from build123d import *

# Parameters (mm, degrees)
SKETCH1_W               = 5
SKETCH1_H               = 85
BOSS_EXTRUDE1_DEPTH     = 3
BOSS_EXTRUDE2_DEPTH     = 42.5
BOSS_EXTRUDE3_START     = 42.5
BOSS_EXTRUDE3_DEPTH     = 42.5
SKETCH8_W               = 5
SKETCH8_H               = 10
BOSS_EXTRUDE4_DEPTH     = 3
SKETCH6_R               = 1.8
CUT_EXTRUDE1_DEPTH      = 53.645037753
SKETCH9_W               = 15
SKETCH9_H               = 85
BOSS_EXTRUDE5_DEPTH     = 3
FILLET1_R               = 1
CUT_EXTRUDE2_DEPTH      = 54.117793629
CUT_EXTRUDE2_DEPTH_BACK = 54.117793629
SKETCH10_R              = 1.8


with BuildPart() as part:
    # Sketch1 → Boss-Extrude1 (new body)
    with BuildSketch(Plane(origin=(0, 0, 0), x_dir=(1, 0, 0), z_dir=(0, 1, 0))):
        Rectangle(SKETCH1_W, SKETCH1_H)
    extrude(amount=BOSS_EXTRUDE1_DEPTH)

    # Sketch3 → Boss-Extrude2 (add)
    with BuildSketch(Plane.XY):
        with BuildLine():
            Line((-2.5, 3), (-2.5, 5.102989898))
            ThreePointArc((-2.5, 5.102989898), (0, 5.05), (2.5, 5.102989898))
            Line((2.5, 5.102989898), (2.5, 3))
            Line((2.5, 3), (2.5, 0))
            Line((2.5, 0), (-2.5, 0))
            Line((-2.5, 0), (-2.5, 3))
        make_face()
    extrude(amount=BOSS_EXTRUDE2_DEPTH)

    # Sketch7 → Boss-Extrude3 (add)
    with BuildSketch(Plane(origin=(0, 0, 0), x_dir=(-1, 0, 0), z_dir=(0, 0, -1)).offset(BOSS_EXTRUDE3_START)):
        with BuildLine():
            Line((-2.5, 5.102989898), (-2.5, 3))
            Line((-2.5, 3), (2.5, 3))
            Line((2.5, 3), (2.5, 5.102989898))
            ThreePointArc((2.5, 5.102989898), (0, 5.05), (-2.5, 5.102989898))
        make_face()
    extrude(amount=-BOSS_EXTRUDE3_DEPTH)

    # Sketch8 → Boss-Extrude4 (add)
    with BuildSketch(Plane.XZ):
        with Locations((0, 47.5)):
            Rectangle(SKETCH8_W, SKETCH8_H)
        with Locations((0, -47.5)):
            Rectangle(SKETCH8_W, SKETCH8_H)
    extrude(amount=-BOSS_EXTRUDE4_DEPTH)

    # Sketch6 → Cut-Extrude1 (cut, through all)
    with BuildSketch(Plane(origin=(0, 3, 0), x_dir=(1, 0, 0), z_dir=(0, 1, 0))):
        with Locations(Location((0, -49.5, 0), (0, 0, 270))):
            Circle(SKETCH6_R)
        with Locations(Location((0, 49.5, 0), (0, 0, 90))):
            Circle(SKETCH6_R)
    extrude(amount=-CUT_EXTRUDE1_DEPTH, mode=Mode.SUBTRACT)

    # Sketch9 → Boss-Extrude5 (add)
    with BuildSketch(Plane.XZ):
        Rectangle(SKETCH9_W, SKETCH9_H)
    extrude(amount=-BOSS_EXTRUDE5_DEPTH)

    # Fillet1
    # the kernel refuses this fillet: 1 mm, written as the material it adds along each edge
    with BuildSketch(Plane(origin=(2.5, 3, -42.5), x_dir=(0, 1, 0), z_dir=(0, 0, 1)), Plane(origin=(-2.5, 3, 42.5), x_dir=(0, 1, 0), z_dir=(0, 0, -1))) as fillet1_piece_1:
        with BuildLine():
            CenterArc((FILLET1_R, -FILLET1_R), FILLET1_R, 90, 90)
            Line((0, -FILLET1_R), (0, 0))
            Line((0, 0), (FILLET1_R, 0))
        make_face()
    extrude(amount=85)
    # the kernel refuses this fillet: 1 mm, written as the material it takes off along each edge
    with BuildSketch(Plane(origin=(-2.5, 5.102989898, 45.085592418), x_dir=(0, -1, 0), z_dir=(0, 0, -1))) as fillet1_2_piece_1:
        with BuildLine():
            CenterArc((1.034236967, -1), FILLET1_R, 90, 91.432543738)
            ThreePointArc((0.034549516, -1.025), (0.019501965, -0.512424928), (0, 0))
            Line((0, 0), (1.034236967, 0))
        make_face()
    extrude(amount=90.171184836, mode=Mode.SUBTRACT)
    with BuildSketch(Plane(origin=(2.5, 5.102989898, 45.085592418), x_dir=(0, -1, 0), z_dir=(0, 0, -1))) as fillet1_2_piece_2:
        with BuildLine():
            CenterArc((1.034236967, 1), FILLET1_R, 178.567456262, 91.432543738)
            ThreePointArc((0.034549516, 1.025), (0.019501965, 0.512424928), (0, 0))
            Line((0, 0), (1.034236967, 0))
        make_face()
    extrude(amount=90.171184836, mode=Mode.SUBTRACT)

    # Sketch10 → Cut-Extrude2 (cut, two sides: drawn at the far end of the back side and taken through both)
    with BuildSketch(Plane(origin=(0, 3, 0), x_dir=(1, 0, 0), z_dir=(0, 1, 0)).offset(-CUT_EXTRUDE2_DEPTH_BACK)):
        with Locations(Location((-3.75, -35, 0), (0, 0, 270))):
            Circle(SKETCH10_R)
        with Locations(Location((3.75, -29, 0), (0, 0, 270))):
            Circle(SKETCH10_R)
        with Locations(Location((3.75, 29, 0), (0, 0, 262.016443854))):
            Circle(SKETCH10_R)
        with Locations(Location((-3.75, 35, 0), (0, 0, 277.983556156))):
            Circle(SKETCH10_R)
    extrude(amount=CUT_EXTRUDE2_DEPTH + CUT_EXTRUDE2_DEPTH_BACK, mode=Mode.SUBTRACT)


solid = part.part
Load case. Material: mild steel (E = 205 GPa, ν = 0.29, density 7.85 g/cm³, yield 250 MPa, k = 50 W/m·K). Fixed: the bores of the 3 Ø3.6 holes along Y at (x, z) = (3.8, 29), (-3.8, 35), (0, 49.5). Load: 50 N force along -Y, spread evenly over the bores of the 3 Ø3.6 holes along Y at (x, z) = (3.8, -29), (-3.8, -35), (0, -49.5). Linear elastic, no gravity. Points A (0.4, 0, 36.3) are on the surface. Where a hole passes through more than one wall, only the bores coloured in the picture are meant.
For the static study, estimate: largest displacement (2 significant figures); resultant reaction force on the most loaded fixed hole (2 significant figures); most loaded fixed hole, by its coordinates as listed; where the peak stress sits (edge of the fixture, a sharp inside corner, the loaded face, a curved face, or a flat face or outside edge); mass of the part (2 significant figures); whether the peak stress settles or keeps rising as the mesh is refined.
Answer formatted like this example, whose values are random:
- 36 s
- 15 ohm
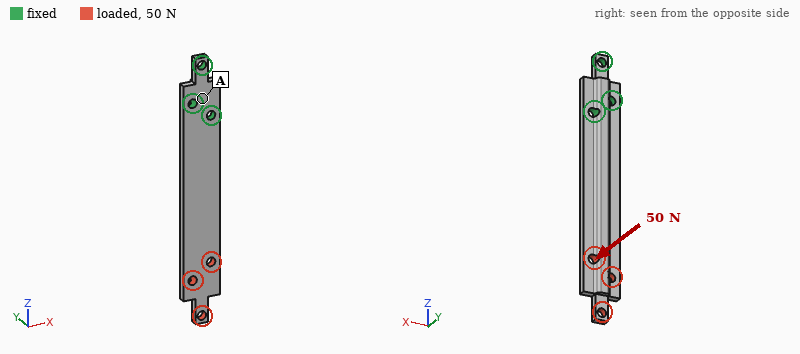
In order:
- 0.37 mm
- 190 N
- (3.8, 29)
- edge of the fixture
- 38 g
- keeps rising
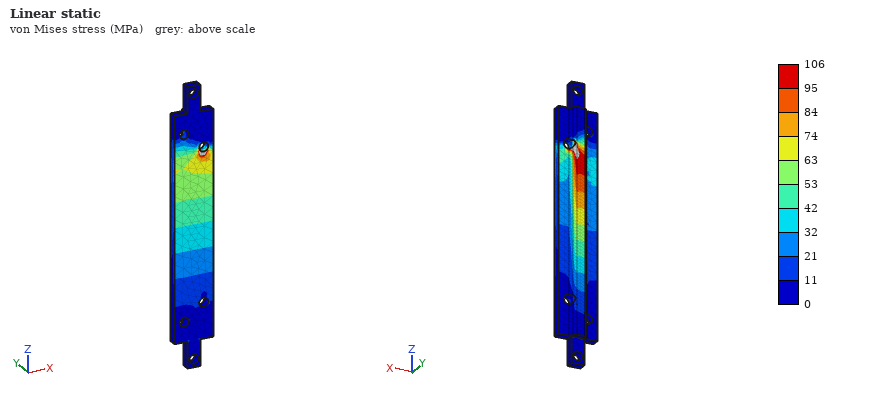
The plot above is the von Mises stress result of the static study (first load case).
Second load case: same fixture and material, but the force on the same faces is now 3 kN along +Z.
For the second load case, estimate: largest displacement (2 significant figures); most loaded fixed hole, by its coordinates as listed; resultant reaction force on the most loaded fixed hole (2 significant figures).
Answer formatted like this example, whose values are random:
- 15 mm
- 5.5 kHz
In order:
- 0.13 mm
- (3.8, 29)
- 1.7 kN
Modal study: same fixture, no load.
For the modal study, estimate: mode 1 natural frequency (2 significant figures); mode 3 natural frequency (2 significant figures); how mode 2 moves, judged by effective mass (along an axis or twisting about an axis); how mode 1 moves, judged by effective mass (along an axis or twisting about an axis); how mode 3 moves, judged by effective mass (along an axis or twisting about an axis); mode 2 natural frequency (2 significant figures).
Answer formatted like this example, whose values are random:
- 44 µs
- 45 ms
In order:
- 670 Hz
- 3900 Hz
- along X
- along Y
- along Y
- 2000 Hz
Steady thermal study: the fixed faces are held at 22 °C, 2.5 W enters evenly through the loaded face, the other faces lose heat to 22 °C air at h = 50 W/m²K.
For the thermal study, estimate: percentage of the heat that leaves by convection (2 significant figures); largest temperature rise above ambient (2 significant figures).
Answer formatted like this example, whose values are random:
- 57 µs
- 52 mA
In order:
- 73 %
- 34 K
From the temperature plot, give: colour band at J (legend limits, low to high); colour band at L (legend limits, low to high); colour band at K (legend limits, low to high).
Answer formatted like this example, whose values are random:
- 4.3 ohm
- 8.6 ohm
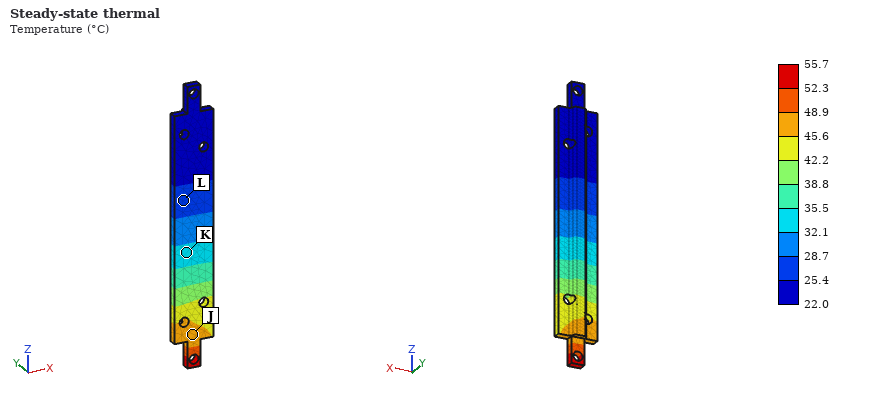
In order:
- 45.6 to 48.9 °C
- 25.4 to 28.7 °C
- 32.1 to 35.5 °C
